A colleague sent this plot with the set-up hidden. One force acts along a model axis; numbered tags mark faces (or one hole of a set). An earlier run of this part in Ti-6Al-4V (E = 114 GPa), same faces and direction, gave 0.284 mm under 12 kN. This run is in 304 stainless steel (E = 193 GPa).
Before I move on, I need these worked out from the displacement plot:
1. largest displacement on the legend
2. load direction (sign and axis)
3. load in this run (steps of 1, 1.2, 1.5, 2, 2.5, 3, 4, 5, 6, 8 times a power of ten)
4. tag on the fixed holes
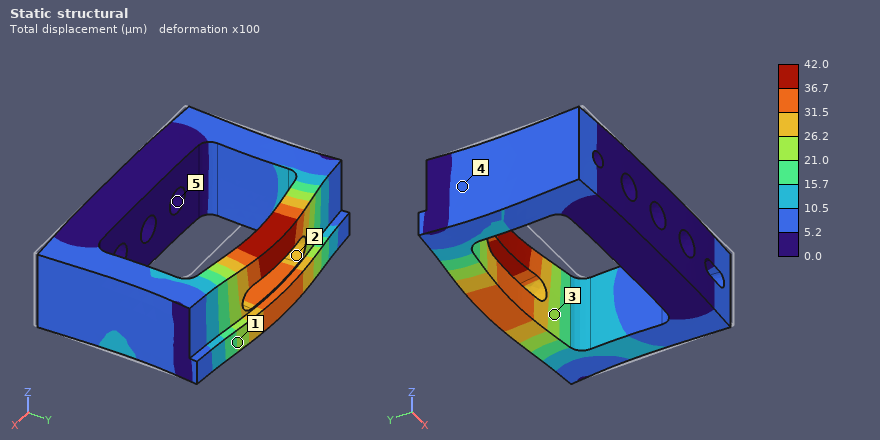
42.0 µm
+Y
3 kN
5
